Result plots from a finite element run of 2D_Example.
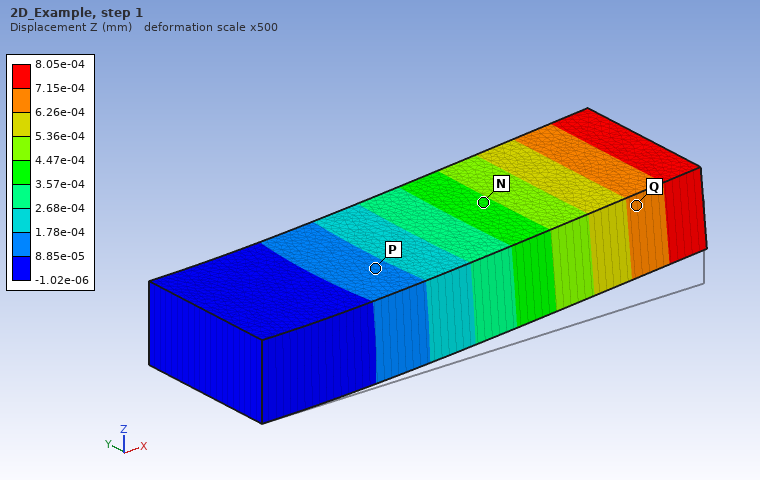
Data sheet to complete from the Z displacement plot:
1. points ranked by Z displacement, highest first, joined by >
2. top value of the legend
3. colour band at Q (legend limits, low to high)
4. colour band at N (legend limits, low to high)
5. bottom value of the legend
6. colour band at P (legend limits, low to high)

Q > N > P
8.05e-04 mm
6.26e-04 to 7.15e-04 mm
3.57e-04 to 4.47e-04 mm
-1.02e-06 mm
8.85e-05 to 1.78e-04 mm
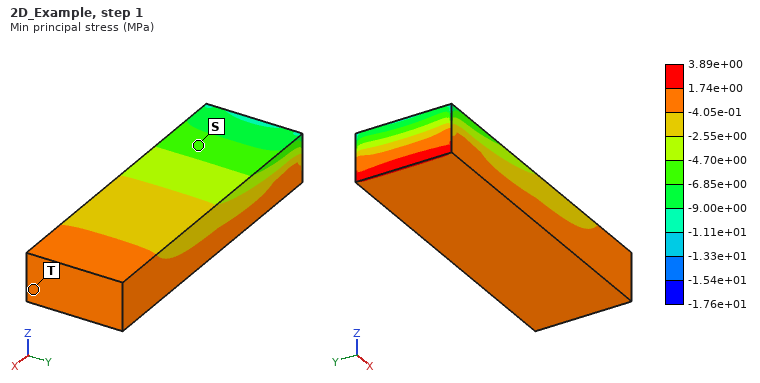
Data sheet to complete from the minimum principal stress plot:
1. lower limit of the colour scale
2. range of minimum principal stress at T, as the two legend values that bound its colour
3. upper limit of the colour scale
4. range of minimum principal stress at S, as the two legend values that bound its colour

-1.76e+01 MPa
-4.05e-01 to 1.74e+00 MPa
3.89e+00 MPa
-6.85e+00 to -4.70e+00 MPa
